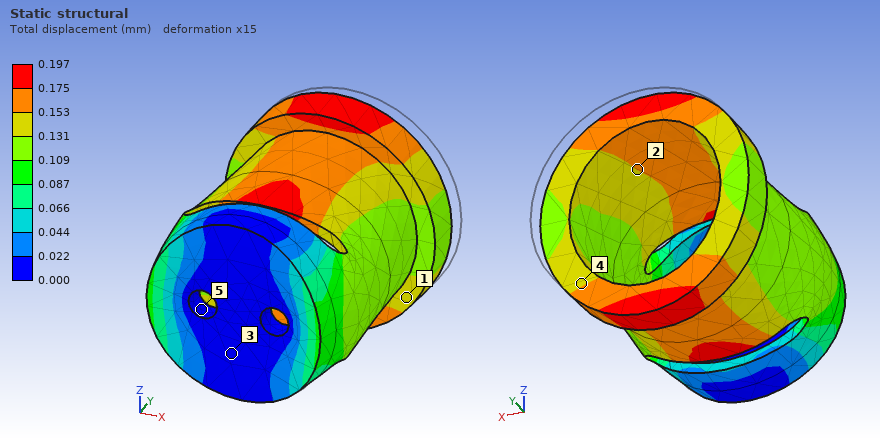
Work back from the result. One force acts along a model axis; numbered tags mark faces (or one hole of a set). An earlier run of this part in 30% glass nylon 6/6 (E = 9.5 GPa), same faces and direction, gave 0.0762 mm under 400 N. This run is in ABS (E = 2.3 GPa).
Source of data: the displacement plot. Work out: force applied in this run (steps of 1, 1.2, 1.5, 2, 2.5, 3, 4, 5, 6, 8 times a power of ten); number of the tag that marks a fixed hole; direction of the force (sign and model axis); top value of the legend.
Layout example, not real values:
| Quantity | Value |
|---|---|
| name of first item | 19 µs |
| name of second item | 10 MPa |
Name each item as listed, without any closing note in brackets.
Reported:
| Quantity | Value |
|---|---|
| force applied in this run | 250 N |
| number of the tag that marks a fixed hole | 5 |
| direction of the force | -Y |
| top value of the legend | 0.197 mm |
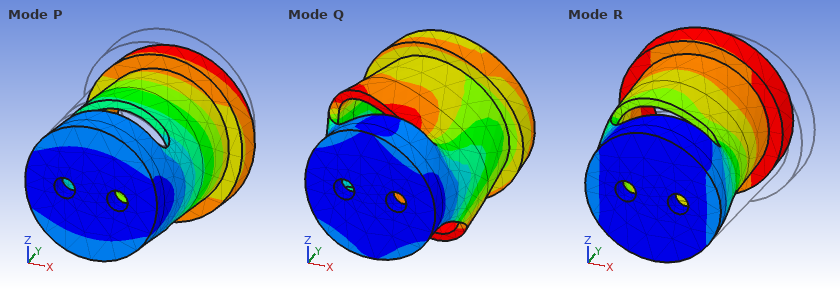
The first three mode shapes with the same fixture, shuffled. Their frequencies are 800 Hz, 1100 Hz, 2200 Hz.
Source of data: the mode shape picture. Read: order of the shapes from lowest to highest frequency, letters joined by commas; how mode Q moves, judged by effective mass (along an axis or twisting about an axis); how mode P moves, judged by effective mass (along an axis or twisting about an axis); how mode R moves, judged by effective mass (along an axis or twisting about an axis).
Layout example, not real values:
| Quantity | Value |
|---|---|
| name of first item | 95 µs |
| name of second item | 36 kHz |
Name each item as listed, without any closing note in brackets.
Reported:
| Quantity | Value |
|---|---|
| order of the shapes from lowest to highest frequency, letters joined by commas | P, R, Q |
| how mode Q moves, judged by effective mass | twisting about Y |
| how mode P moves, judged by effective mass | along Z |
| how mode R moves, judged by effective mass | along X |
